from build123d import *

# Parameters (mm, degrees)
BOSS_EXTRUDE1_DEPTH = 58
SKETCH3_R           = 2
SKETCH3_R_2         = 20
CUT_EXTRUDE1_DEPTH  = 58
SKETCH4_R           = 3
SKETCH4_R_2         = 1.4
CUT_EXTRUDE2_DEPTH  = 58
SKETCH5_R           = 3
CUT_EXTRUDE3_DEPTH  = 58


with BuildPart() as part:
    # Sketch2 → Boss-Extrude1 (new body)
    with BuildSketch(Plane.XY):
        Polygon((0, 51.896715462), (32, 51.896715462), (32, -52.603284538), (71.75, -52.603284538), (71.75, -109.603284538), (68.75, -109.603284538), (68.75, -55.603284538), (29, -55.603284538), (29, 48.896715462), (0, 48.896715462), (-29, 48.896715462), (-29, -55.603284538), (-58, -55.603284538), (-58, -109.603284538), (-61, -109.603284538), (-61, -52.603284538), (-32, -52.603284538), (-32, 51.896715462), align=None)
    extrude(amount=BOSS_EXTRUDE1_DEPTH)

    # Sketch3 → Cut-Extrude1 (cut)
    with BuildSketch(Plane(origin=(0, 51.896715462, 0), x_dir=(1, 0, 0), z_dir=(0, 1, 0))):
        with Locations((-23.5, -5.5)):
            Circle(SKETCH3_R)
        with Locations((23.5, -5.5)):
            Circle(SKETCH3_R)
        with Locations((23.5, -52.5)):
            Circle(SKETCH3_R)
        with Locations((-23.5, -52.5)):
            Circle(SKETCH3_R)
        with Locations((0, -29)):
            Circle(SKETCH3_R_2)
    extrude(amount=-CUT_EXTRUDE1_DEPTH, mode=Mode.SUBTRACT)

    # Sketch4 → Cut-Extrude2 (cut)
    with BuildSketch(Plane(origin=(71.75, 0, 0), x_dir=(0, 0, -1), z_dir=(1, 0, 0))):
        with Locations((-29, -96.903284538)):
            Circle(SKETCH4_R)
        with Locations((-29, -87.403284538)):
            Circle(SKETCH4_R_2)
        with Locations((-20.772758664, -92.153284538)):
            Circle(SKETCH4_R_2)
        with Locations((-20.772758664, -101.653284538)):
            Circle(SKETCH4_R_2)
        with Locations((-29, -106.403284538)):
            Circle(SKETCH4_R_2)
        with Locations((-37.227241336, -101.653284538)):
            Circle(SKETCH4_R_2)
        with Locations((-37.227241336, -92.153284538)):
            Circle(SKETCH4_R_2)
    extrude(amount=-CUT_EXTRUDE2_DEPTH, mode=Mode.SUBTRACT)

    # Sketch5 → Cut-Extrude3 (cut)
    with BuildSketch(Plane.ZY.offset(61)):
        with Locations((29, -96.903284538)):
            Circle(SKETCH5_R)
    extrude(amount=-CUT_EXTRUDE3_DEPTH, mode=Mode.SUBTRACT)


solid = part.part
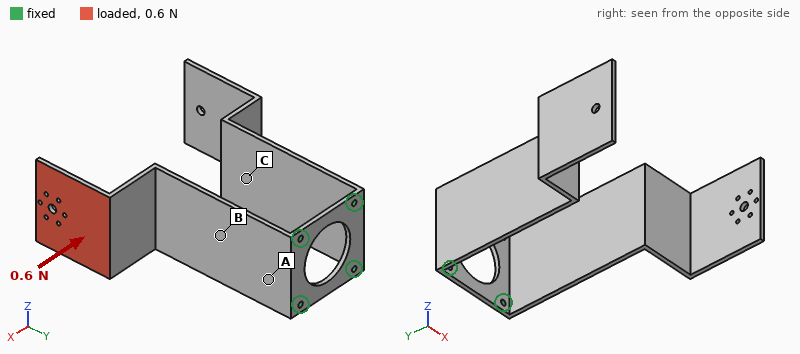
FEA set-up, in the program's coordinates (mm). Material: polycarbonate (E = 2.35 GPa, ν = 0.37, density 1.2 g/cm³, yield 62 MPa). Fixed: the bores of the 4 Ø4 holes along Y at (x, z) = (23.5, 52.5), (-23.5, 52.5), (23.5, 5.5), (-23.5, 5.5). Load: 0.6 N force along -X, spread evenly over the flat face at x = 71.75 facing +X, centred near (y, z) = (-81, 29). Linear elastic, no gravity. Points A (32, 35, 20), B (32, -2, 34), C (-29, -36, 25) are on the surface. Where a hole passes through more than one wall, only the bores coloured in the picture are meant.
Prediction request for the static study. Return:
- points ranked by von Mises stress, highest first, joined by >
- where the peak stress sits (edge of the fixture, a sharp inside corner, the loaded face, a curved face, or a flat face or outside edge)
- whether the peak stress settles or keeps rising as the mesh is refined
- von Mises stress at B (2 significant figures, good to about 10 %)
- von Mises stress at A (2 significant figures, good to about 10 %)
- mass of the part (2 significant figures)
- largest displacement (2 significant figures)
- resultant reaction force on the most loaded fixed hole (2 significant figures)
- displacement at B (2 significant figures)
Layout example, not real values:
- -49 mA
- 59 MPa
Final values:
- A > B > C
- edge of the fixture
- keeps rising
- 0.51 MPa
- 0.70 MPa
- 89 g
- 2.4 mm
- 0.48 N
- 0.40 mm
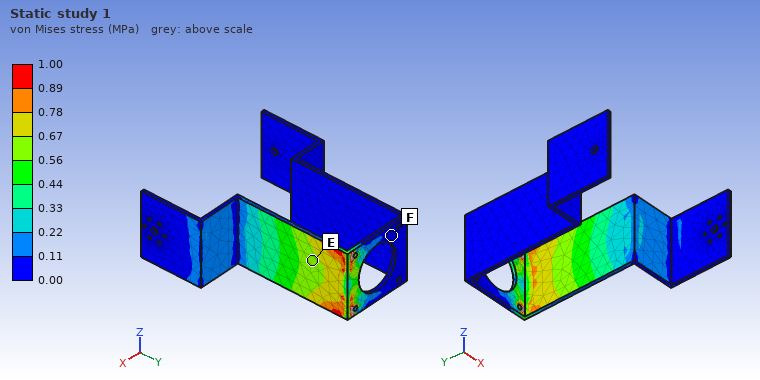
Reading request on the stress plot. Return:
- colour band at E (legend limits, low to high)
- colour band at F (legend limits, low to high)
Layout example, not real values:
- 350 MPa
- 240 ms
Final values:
- 0.56 to 0.67 MPa
- 0.00 to 0.11 MPa
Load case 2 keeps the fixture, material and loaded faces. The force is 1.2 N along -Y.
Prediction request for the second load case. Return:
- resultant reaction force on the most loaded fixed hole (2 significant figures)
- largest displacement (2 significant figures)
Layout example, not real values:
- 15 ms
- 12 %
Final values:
- 0.67 N
- 2.3 mm
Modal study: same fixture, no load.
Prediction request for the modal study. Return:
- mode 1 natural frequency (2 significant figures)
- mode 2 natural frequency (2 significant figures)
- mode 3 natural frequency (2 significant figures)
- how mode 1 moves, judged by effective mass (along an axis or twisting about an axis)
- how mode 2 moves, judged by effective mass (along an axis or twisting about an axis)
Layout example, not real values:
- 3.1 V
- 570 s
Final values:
- 21 Hz
- 22 Hz
- 67 Hz
- along X
- along X
